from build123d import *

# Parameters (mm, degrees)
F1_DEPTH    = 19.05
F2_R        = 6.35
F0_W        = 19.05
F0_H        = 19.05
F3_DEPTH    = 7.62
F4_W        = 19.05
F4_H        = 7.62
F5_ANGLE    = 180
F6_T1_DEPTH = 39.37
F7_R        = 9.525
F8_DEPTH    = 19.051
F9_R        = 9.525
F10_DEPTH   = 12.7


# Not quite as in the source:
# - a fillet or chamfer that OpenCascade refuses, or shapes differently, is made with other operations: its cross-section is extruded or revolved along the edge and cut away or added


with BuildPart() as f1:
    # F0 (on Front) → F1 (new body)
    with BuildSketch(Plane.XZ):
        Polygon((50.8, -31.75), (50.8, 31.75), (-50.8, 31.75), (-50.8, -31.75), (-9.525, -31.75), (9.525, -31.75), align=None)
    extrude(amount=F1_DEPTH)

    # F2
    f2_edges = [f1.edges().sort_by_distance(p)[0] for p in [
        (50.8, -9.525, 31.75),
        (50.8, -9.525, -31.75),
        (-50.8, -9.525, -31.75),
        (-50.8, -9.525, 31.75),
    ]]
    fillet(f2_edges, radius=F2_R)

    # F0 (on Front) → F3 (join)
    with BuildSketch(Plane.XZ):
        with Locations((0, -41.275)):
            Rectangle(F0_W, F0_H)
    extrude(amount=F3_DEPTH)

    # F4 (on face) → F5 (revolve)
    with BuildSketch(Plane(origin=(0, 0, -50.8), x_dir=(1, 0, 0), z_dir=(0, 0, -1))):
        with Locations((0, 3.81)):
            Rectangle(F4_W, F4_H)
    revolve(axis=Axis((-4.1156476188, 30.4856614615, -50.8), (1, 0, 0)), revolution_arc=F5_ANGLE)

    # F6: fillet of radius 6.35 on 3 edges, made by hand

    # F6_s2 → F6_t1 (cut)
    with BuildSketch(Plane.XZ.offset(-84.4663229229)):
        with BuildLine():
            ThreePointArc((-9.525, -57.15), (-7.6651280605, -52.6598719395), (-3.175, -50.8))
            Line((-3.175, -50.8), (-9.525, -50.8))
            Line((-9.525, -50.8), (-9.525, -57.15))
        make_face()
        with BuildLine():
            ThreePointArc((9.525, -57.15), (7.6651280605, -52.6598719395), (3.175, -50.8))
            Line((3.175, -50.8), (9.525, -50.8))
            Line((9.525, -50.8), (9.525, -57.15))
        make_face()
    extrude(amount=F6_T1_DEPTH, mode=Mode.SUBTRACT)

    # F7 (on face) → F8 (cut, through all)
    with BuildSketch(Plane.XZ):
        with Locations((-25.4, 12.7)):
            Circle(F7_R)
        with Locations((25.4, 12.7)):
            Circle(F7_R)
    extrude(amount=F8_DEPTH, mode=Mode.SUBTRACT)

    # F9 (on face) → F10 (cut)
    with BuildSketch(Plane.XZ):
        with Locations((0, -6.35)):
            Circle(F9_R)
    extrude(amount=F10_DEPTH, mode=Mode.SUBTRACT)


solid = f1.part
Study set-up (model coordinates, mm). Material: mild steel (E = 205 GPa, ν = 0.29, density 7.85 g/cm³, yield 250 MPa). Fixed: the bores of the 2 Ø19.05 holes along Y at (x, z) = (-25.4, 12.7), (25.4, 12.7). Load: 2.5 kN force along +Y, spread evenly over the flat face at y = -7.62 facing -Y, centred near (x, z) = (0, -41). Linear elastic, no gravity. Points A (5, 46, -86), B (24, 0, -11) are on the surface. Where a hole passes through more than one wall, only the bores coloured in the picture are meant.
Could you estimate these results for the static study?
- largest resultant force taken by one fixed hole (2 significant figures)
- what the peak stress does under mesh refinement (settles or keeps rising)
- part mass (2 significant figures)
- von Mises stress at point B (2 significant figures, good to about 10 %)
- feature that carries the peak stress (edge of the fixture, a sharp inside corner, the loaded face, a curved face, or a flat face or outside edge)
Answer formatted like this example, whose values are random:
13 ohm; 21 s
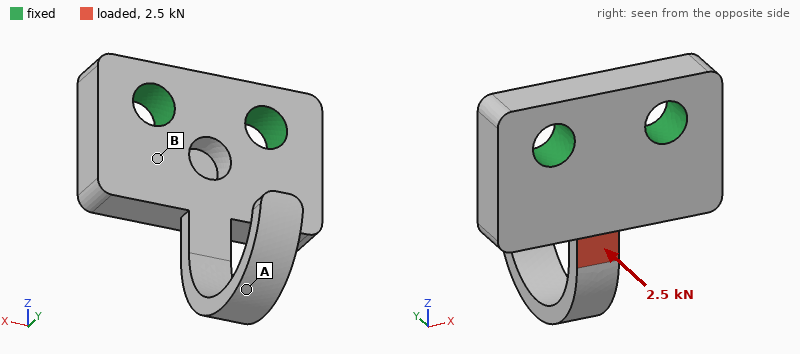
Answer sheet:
1.3 kN; keeps rising; 990 g; 17 MPa; a sharp inside corner
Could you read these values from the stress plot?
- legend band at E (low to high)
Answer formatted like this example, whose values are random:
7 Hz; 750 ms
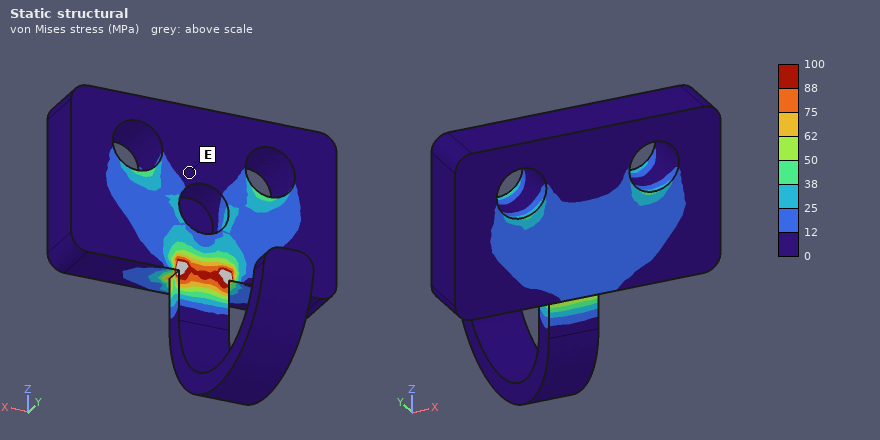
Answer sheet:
0 to 12 MPa
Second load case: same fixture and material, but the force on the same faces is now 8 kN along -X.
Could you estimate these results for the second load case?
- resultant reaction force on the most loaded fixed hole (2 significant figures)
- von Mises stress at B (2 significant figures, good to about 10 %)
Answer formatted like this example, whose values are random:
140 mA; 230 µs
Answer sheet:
7.4 kN; 19 MPa
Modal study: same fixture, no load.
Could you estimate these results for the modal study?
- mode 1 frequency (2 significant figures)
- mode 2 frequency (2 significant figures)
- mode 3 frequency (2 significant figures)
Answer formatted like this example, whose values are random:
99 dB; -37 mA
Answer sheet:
490 Hz; 650 Hz; 1300 Hz
